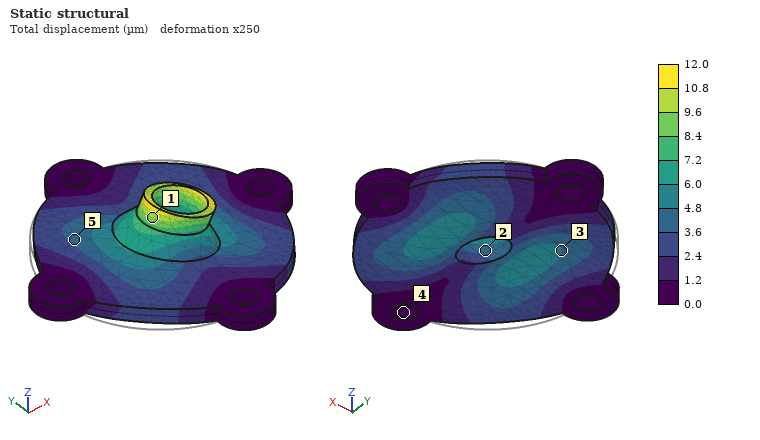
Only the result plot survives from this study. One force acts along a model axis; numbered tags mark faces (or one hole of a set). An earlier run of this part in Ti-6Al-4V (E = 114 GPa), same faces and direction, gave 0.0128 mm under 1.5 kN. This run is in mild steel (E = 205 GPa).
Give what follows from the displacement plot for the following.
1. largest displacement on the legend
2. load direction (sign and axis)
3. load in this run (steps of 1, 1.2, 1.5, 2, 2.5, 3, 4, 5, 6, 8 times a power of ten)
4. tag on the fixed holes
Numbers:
12.0 µm
+X
2.5 kN
4
